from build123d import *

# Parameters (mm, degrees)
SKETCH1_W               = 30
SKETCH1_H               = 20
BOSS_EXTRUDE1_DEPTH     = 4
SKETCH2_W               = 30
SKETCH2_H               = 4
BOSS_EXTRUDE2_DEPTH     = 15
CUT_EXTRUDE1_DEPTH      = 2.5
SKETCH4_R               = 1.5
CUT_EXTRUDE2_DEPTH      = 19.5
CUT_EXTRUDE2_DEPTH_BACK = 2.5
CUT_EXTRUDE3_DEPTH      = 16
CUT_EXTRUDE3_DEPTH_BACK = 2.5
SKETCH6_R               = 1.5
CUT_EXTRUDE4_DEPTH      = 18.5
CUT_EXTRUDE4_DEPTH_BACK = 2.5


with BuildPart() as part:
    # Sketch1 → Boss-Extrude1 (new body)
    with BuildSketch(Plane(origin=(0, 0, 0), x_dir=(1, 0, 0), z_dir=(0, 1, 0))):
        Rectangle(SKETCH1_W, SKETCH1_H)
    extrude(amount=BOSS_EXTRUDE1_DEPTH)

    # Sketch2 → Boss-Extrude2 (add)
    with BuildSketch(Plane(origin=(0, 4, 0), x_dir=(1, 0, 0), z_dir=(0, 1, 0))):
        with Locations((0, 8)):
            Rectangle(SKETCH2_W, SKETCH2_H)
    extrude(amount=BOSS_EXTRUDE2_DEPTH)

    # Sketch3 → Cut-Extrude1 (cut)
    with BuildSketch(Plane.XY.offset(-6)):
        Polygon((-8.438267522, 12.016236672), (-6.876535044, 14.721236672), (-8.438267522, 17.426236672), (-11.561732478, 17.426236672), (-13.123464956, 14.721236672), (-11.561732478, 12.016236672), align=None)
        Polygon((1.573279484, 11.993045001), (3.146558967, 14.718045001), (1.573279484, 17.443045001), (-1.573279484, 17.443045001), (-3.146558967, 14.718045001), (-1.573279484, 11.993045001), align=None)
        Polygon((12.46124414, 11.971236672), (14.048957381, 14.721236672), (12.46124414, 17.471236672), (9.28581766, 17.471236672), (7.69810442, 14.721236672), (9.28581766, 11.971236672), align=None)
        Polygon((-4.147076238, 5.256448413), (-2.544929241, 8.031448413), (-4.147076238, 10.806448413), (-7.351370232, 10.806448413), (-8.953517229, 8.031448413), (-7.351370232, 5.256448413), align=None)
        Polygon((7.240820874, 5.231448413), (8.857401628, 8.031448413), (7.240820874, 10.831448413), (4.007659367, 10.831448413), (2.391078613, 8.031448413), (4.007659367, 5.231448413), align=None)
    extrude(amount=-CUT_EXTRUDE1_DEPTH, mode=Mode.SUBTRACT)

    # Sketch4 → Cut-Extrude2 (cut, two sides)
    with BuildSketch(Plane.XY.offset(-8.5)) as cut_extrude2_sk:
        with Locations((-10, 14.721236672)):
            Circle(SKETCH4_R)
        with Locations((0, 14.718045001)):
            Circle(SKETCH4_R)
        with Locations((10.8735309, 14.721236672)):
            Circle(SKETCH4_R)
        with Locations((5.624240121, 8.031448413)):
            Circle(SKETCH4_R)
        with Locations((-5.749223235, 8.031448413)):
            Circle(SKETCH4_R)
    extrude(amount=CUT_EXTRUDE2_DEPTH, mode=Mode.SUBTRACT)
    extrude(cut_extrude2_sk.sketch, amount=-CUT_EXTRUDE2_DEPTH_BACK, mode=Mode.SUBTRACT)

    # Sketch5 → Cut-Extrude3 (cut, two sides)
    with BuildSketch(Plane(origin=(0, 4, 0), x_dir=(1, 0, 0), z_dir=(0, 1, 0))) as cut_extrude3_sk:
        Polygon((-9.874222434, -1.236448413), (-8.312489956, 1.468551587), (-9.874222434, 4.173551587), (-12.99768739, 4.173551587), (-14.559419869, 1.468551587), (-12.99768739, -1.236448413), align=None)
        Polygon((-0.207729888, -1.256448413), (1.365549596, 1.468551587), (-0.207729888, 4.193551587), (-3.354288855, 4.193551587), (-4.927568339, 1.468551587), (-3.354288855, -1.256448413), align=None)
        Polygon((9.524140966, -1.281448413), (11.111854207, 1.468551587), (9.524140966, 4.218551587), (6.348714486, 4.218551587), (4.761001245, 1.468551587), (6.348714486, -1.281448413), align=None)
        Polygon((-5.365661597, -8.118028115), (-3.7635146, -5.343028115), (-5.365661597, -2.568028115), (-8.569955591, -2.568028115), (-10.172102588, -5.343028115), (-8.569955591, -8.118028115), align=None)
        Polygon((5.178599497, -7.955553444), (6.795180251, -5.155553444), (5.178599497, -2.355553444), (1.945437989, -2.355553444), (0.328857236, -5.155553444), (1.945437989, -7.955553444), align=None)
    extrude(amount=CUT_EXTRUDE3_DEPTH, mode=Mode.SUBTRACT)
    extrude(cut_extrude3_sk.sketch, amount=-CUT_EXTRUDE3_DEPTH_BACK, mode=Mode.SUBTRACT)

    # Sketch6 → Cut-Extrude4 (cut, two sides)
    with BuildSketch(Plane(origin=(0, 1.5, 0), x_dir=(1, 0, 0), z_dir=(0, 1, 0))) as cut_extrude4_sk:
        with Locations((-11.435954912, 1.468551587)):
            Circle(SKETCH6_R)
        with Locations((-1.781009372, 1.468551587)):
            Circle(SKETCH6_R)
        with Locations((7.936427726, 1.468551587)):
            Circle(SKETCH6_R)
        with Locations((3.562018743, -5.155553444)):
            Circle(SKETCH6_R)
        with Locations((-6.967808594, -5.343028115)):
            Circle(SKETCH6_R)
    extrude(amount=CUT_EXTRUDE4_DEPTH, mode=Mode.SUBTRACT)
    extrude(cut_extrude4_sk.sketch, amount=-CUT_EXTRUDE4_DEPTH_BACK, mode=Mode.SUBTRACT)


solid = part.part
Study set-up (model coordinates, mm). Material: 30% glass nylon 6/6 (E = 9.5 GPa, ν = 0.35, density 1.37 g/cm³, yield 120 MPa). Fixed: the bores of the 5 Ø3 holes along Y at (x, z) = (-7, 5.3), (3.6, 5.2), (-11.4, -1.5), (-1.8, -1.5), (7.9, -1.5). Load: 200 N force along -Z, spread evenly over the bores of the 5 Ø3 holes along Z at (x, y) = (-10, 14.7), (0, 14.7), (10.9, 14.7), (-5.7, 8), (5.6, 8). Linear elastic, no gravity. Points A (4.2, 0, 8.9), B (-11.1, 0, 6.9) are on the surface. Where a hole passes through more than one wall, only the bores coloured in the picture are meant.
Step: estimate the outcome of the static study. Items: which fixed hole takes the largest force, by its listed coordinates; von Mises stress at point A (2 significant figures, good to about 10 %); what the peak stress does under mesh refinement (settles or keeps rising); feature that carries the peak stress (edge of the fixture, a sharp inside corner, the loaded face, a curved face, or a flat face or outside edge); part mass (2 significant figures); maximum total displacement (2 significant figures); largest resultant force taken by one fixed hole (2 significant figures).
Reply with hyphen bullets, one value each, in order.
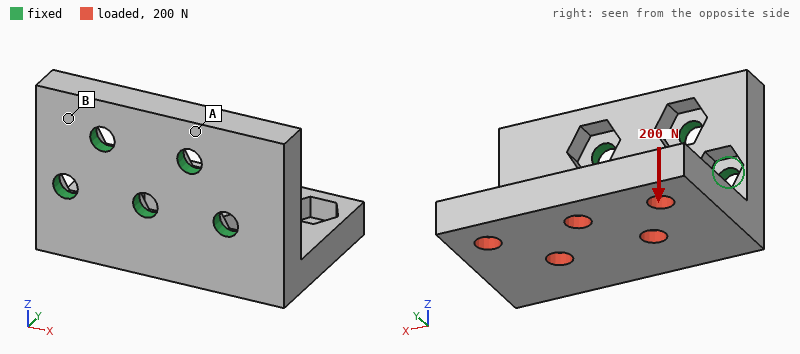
- (3.6, 5.2)
- 12 MPa
- keeps rising
- edge of the fixture
- 4.7 g
- 0.39 mm
- 170 N
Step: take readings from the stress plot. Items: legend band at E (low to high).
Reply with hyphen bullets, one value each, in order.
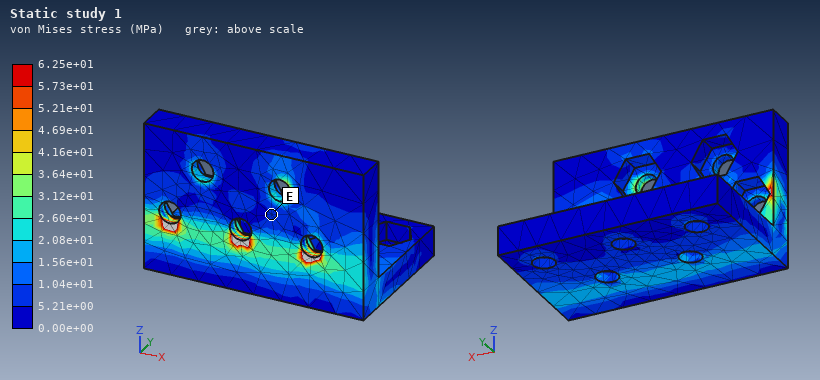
- 5.21e+00 to 1.04e+01 MPa
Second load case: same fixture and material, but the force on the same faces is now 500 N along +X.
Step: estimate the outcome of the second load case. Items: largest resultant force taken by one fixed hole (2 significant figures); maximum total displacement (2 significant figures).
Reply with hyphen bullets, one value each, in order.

- 390 N
- 0.17 mm
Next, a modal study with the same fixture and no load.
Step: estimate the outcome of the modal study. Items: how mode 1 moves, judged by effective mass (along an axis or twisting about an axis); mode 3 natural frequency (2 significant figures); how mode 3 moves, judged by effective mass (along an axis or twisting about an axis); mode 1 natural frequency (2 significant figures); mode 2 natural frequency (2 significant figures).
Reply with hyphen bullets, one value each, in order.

- along Z
- 8800 Hz
- along X
- 3100 Hz
- 5500 Hz
